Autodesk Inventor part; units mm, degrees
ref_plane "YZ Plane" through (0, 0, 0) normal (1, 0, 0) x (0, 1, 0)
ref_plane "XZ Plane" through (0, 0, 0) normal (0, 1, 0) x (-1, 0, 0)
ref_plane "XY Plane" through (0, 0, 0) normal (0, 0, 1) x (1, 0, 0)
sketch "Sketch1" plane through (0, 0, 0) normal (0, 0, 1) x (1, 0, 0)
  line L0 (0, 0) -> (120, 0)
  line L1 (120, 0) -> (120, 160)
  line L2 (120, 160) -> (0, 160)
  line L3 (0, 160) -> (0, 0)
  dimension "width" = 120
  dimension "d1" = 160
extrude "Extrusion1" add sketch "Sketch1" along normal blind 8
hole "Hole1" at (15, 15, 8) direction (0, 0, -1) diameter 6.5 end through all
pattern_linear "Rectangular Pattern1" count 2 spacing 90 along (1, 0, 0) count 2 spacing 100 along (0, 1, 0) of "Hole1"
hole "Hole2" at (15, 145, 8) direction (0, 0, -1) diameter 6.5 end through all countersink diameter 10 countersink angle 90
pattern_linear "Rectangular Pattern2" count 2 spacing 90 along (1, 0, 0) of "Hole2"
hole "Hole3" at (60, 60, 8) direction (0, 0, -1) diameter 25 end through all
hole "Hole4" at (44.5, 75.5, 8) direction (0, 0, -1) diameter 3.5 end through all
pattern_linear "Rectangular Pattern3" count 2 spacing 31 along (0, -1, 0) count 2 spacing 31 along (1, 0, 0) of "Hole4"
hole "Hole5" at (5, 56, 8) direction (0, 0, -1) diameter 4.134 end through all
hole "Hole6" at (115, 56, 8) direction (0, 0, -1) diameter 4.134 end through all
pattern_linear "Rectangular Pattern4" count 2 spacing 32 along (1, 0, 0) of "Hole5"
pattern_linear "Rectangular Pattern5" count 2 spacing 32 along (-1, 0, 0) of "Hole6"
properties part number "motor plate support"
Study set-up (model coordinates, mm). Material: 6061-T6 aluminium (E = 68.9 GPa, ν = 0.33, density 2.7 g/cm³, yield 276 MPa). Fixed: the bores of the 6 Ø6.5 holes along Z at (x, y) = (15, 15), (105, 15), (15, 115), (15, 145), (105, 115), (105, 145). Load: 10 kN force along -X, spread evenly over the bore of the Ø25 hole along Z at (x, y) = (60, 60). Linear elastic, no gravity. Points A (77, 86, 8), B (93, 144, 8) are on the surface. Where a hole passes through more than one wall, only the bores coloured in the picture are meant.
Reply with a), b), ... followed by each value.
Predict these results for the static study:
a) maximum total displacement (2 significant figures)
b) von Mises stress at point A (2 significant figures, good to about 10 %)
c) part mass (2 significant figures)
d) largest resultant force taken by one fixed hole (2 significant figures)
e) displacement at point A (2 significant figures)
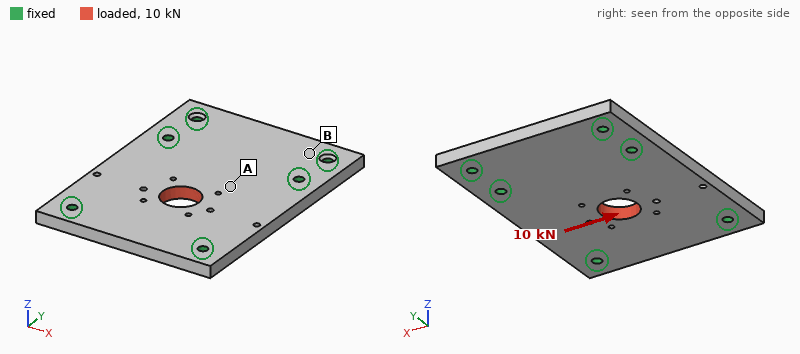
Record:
a) 15 µm
b) 12 MPa
c) 400 g
d) 2.9 kN
e) 8.3 µm
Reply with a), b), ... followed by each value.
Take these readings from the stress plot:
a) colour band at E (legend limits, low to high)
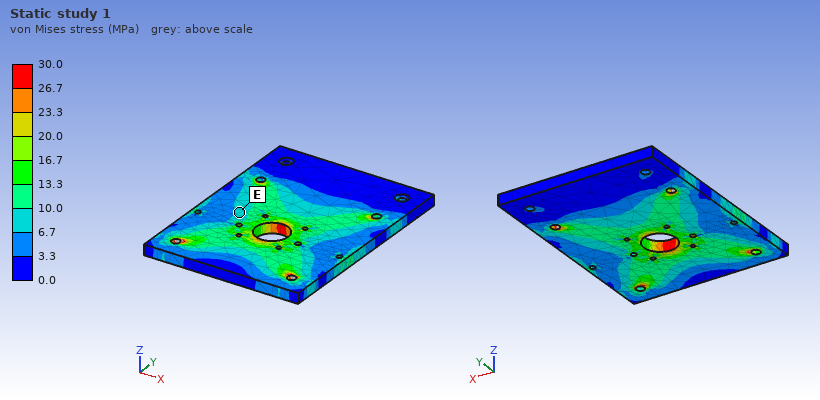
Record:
a) 6.7 to 10.0 MPa
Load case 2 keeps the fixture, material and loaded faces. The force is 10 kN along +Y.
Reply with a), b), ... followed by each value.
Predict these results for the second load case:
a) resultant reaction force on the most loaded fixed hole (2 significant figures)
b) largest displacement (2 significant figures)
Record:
a) 2.5 kN
b) 13 µm
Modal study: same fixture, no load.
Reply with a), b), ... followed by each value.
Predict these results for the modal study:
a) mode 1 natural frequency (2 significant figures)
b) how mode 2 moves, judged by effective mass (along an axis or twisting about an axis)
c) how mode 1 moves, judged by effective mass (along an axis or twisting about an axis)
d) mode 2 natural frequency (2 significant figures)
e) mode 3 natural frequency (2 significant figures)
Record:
a) 3100 Hz
b) twisting about Y
c) along Z
d) 4400 Hz
e) 4800 Hz
